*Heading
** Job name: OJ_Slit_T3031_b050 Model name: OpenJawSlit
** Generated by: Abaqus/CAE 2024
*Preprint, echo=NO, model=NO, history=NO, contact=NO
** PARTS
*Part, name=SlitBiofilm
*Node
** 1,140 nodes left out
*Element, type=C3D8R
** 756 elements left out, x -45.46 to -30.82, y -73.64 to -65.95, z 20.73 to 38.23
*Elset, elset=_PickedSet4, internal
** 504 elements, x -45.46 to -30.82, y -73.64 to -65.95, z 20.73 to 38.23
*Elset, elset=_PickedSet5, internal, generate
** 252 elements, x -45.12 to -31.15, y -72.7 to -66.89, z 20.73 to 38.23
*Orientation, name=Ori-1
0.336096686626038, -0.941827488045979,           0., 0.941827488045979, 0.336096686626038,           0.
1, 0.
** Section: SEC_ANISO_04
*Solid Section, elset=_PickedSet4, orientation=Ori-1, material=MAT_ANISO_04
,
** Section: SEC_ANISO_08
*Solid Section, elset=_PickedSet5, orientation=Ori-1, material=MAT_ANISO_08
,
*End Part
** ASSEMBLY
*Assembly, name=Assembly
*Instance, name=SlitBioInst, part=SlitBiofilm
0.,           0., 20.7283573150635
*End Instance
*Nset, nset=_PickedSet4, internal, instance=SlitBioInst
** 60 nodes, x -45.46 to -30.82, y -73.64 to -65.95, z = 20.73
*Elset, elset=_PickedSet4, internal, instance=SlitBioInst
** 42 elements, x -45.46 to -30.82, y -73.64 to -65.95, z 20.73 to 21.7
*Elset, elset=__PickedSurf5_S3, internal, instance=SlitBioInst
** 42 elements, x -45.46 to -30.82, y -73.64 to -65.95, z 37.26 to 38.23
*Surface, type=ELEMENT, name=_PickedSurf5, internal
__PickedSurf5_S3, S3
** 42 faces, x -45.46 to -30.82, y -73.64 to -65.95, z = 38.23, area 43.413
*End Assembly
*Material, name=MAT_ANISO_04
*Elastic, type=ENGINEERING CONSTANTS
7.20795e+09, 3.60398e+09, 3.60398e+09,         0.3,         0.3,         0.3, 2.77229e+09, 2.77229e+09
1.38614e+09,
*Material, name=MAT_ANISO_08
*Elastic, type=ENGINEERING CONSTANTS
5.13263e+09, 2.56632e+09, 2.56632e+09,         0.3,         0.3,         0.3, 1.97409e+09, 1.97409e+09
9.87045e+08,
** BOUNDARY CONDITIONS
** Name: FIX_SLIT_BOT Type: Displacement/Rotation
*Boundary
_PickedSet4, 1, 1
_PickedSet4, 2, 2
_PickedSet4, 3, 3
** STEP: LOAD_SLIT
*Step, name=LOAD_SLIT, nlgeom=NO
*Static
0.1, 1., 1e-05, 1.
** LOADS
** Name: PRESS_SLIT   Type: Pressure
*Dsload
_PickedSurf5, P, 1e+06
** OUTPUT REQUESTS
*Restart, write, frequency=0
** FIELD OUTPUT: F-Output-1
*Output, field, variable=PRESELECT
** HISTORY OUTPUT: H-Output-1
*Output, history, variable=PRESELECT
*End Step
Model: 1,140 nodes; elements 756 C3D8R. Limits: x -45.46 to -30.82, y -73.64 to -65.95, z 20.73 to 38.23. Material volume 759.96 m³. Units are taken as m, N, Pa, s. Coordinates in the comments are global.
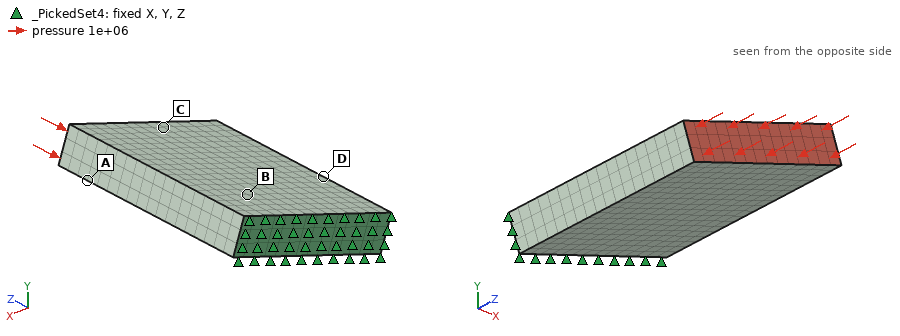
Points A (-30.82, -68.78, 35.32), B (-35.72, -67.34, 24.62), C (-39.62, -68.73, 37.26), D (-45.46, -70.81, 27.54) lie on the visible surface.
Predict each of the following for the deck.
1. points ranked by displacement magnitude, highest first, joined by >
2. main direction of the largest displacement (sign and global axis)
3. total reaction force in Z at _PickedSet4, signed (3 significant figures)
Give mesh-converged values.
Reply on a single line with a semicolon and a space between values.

C > A > D > B; -Z; 4.34e+07 N
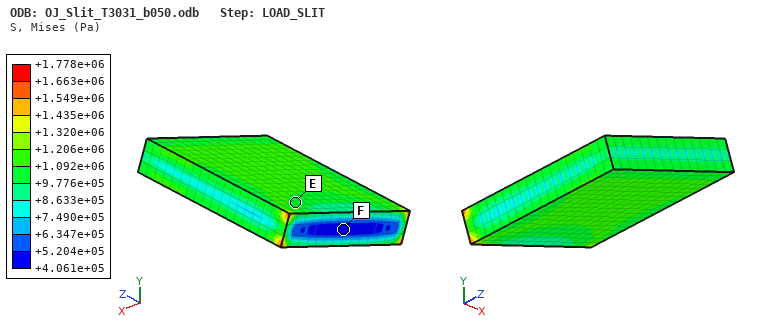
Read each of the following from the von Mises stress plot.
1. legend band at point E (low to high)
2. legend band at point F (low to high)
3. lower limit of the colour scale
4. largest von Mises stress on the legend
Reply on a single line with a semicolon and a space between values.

+9.776e+05 to +1.092e+06 Pa; +4.061e+05 to +5.204e+05 Pa; +4.061e+05 Pa; +1.778e+06 Pa
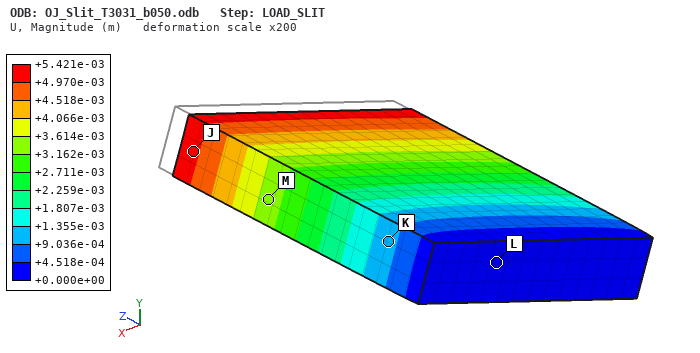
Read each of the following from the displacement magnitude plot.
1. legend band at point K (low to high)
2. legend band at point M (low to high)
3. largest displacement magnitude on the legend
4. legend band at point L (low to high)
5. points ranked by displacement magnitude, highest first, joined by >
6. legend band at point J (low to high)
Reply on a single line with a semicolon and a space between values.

+9.036e-04 to +1.355e-03 m; +3.162e-03 to +3.614e-03 m; +5.421e-03 m; +0.000e+00 to +4.518e-04 m; J > M > K > L; +4.970e-03 to +5.421e-03 m
